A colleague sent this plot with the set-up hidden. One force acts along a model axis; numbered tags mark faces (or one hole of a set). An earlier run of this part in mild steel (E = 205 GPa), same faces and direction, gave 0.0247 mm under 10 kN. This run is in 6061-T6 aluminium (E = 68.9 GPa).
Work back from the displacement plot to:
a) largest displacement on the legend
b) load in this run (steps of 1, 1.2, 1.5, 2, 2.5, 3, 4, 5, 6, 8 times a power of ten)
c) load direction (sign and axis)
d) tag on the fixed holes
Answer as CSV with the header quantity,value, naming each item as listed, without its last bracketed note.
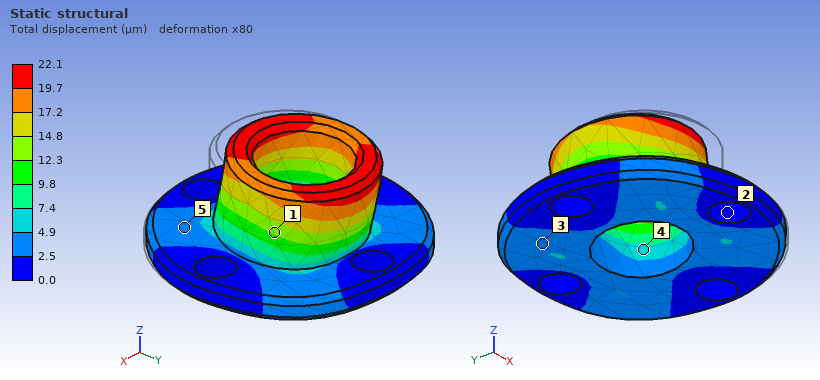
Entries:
quantity,value
largest displacement on the legend,22.1 µm
load in this run,3 kN
load direction,+Y
tag on the fixed holes,2
